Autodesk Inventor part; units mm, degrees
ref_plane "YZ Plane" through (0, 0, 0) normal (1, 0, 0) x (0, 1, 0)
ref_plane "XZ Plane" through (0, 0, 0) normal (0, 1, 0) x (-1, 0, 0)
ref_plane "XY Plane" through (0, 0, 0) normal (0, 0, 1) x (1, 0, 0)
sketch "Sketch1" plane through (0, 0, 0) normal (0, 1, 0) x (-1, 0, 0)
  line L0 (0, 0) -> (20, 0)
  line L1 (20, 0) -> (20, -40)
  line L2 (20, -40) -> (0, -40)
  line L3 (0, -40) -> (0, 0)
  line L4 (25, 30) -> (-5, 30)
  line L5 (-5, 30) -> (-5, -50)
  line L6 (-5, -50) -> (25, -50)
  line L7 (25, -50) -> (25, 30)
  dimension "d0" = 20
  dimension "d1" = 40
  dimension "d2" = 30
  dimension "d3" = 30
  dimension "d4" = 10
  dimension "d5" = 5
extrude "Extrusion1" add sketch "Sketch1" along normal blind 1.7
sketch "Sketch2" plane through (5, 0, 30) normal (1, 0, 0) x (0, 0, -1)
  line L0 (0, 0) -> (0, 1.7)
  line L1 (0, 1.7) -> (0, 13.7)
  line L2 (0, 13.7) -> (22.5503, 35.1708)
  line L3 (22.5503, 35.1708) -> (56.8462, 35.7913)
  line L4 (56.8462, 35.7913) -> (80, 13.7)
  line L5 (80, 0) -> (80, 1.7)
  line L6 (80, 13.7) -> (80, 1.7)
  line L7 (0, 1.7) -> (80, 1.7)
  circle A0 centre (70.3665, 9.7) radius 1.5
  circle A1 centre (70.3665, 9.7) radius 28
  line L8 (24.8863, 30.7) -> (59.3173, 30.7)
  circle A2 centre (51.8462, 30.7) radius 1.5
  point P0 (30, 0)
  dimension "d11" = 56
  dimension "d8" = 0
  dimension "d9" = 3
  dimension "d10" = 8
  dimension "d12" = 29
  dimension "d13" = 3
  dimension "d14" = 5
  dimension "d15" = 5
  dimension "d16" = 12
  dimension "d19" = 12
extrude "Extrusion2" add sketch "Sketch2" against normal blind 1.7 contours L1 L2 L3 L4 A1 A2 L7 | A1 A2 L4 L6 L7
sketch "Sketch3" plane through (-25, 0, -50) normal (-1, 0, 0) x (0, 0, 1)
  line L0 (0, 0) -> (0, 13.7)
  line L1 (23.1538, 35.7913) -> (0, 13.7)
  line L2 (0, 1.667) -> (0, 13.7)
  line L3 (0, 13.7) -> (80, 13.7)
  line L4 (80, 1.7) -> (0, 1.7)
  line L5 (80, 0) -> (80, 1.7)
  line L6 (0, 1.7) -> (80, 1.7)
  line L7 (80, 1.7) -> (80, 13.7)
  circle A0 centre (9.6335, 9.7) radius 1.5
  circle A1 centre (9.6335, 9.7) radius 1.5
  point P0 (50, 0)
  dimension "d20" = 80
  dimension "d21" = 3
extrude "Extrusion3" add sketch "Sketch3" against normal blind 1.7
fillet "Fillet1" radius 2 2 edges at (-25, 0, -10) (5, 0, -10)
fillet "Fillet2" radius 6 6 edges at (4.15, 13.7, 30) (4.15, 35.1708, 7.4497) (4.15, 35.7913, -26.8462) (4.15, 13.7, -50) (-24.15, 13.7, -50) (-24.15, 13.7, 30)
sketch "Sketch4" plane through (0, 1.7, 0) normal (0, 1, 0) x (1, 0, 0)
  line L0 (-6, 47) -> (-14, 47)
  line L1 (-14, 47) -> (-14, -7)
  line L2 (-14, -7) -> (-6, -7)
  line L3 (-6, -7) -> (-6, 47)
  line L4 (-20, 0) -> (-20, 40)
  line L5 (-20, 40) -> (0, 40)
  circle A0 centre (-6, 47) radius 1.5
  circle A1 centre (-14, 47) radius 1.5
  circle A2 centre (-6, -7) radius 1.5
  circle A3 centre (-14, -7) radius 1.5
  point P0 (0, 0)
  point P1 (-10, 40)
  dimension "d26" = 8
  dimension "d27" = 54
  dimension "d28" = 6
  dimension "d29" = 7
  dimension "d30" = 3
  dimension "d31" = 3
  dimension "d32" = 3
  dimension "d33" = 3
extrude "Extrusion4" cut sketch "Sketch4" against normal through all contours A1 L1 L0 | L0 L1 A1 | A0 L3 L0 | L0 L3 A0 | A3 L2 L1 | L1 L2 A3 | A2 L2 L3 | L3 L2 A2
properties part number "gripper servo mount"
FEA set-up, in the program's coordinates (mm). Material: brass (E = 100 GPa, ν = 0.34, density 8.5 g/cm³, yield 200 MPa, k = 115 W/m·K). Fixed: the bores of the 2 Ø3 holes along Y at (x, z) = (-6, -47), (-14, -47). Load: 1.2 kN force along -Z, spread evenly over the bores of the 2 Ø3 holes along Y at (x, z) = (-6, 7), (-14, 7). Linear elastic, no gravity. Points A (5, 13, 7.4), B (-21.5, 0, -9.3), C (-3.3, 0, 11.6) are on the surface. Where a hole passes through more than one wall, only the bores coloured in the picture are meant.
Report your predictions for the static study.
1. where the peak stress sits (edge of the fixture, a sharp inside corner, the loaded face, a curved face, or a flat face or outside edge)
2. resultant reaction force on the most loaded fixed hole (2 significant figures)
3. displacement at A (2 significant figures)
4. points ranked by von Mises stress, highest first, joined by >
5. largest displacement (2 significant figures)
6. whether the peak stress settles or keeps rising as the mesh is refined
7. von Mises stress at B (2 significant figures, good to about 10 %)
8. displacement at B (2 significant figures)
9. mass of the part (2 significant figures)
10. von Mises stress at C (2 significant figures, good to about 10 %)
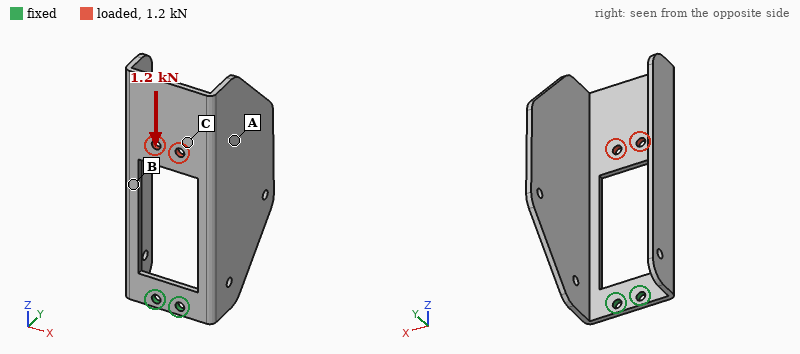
edge of the fixture
790 N
54 µm
B > C > A
93 µm
keeps rising
58 MPa
43 µm
67 g
35 MPa
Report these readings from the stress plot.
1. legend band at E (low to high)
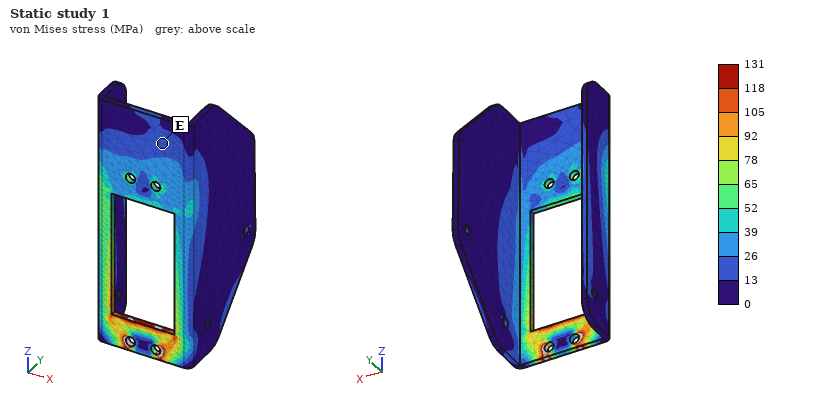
13 to 26 MPa
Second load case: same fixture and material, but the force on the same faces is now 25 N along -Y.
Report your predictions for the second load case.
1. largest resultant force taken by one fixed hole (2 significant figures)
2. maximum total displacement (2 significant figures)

19 N
0.67 mm
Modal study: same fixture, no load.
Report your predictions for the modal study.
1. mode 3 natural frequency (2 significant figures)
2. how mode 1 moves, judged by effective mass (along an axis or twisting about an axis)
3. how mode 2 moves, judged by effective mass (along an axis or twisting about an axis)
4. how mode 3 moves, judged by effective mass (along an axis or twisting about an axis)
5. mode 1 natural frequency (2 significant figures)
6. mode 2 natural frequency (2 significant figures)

600 Hz
along Y
along X
along X
160 Hz
270 Hz
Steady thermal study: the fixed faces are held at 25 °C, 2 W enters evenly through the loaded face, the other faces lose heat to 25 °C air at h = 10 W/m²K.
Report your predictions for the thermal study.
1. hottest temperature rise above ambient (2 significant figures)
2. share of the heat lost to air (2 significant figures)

15 K
41 %
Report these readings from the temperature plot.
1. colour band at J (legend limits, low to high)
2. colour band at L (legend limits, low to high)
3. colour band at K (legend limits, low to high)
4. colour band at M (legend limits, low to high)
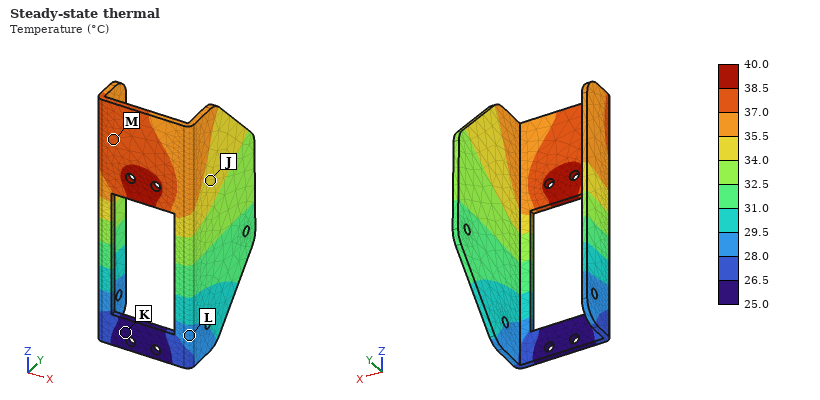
34.0 to 35.5 °C
28.0 to 29.5 °C
25.0 to 26.5 °C
37.0 to 38.5 °C
